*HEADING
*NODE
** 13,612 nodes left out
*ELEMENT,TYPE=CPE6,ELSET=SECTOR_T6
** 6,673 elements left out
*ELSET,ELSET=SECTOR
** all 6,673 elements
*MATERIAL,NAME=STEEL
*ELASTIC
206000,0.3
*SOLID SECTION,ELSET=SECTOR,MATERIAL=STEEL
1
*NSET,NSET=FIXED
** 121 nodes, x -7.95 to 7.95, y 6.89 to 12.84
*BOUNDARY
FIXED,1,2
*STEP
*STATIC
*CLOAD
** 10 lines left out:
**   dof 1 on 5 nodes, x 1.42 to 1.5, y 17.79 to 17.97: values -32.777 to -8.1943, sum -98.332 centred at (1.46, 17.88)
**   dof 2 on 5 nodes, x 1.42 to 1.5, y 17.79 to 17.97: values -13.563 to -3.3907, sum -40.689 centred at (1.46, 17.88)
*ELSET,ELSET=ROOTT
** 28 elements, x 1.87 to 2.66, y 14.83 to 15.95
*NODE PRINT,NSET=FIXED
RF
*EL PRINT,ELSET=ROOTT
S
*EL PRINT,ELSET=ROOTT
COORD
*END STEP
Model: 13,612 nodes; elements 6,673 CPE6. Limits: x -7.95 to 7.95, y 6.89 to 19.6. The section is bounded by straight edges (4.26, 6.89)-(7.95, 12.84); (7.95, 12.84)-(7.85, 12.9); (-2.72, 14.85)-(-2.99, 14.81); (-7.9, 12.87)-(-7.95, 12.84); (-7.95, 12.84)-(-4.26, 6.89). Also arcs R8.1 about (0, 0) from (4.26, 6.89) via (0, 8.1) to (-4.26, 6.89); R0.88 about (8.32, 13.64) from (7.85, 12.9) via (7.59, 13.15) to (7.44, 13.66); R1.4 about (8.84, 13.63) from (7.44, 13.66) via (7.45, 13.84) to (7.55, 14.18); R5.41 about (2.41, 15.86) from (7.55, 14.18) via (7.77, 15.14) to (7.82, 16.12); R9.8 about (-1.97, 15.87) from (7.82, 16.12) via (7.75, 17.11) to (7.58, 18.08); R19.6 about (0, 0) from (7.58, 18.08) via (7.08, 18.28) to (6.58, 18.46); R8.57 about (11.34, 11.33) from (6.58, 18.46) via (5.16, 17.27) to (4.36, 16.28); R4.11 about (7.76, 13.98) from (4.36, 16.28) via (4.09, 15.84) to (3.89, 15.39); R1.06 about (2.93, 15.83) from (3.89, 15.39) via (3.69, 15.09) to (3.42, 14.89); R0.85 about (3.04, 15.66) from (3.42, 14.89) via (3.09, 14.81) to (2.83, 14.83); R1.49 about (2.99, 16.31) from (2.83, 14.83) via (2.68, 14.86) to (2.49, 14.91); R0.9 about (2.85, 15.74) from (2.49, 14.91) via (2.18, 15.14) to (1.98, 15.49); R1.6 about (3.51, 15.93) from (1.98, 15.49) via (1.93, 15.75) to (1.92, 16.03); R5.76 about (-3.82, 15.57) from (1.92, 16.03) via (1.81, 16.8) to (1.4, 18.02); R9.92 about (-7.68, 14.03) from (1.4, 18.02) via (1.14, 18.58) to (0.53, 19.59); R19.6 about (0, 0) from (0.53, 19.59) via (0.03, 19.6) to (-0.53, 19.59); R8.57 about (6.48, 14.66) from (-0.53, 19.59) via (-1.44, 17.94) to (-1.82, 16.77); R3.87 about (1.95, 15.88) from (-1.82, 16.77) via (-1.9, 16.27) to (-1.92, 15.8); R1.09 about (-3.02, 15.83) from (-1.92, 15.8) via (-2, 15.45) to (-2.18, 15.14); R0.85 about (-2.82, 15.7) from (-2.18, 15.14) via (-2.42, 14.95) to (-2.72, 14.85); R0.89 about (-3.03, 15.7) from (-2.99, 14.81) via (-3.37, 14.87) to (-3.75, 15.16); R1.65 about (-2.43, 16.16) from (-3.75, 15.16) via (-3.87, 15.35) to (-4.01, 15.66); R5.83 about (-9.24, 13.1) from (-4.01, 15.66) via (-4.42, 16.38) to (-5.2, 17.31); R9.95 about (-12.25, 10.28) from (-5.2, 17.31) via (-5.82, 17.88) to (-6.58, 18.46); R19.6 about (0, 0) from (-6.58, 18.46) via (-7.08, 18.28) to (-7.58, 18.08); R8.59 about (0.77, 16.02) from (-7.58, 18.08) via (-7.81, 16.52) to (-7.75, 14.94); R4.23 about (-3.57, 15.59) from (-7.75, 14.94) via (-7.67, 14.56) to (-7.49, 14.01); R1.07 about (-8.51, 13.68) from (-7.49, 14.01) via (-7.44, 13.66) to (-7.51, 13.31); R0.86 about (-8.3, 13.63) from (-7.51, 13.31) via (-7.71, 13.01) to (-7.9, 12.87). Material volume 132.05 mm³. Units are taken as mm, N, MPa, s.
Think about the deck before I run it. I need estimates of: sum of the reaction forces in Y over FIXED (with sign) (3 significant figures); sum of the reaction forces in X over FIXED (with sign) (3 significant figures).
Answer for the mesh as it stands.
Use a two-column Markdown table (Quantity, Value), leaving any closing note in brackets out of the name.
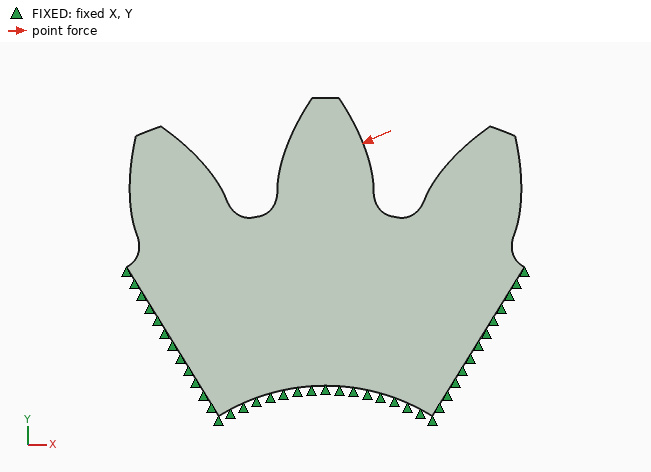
| Quantity | Value |
|---|---|
| sum of the reaction forces in Y over FIXED (with sign) | 40.7 N |
| sum of the reaction forces in X over FIXED (with sign) | 98.3 N |
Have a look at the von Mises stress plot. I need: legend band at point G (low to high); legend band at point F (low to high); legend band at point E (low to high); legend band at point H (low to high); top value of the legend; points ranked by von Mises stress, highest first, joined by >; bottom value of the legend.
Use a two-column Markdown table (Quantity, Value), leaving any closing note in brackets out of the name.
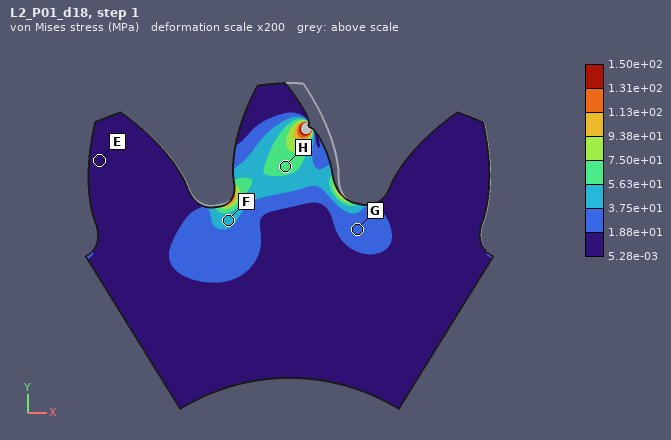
| Quantity | Value |
|---|---|
| legend band at point G | 1.88e+01 to 3.75e+01 MPa |
| legend band at point F | 3.75e+01 to 5.63e+01 MPa |
| legend band at point E | 5.28e-03 to 1.88e+01 MPa |
| legend band at point H | 5.63e+01 to 7.50e+01 MPa |
| top value of the legend | 1.50e+02 MPa |
| points ranked by von Mises stress, highest first, joined by > | H > F > G > E |
| bottom value of the legend | 5.28e-03 MPa |
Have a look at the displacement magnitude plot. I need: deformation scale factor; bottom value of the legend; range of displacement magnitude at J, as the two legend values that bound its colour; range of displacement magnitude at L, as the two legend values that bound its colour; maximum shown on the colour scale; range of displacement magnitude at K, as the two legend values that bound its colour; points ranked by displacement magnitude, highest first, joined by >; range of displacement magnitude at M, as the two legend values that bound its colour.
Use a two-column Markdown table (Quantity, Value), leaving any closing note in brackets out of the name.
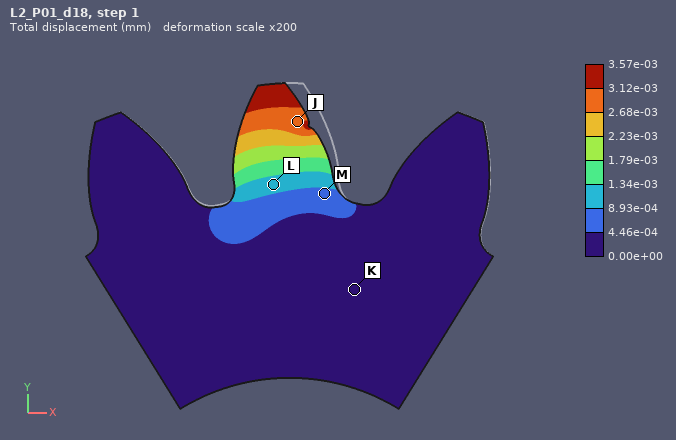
| Quantity | Value |
|---|---|
| deformation scale factor | 200 |
| bottom value of the legend | 0.00e+00 mm |
| range of displacement magnitude at J, as the two legend values that bound its colour | 2.68e-03 to 3.12e-03 mm |
| range of displacement magnitude at L, as the two legend values that bound its colour | 8.93e-04 to 1.34e-03 mm |
| maximum shown on the colour scale | 3.57e-03 mm |
| range of displacement magnitude at K, as the two legend values that bound its colour | 0.00e+00 to 4.46e-04 mm |
| points ranked by displacement magnitude, highest first, joined by > | J > L > M > K |
| range of displacement magnitude at M, as the two legend values that bound its colour | 4.46e-04 to 8.93e-04 mm |
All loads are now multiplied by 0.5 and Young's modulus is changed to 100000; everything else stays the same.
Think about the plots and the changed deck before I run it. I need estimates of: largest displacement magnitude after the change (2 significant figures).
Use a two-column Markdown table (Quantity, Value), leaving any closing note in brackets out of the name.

| Quantity | Value |
|---|---|
| largest displacement magnitude after the change | 0.0037 mm |
